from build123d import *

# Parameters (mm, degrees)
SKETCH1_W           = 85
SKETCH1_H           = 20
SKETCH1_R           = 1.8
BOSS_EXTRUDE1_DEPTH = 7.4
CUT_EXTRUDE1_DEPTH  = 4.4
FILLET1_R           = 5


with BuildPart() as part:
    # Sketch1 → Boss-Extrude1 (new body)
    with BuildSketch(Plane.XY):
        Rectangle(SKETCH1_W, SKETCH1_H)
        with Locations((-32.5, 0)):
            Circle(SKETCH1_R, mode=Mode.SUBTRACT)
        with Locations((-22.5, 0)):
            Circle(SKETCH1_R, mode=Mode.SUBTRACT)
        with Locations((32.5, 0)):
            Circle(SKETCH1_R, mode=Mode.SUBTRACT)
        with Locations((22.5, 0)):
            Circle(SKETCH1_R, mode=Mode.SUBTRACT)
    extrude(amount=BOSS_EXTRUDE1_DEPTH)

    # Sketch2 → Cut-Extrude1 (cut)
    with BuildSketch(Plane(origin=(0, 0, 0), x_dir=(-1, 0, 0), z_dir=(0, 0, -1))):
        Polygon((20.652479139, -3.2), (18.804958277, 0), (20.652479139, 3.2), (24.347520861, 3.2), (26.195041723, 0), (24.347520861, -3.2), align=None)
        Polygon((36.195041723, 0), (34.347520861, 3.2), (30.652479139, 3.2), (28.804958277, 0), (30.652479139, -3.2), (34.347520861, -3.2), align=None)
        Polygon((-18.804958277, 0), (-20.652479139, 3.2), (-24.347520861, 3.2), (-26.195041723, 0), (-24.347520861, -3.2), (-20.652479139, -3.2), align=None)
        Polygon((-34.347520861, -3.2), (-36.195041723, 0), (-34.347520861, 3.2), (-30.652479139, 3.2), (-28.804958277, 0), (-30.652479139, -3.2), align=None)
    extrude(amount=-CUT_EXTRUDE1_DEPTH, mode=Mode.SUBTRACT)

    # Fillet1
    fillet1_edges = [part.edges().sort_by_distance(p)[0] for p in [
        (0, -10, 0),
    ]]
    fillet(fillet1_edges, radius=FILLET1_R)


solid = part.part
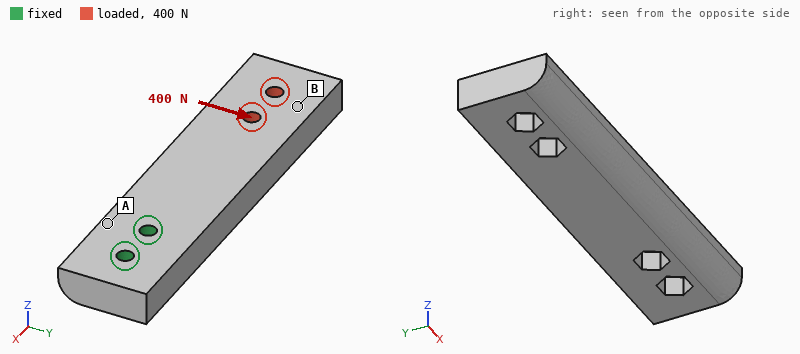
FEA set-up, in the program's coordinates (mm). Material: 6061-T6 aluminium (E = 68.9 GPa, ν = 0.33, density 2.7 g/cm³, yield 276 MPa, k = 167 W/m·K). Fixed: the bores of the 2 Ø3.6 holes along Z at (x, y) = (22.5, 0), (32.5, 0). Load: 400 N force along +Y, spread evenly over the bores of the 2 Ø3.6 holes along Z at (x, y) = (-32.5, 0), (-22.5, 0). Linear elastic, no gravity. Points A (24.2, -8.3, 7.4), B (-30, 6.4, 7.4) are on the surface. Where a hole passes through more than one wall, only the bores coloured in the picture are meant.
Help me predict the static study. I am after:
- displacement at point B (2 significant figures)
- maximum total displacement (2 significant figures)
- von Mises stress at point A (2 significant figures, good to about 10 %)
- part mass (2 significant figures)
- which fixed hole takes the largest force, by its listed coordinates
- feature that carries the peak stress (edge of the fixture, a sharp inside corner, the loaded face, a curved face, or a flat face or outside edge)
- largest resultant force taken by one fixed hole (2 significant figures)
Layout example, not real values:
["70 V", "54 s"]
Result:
["0.13 mm", "0.17 mm", "31 MPa", "31 g", "(22.5, 0)", "edge of the fixture", "1.8 kN"]
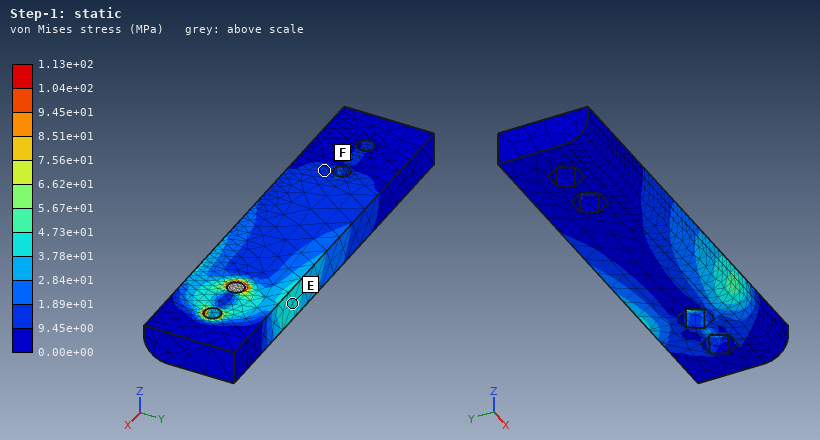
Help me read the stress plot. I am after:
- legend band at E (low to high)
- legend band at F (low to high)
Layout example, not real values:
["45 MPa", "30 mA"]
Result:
["3.78e+01 to 4.73e+01 MPa", "9.45e+00 to 1.89e+01 MPa"]
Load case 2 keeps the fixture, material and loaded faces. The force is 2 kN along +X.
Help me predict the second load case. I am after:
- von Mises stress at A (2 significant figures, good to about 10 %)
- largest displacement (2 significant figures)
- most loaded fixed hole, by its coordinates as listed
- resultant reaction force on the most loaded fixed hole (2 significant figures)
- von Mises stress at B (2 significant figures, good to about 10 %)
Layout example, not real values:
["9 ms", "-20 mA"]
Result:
["18 MPa", "0.19 mm", "(22.5, 0)", "1.5 kN", "17 MPa"]
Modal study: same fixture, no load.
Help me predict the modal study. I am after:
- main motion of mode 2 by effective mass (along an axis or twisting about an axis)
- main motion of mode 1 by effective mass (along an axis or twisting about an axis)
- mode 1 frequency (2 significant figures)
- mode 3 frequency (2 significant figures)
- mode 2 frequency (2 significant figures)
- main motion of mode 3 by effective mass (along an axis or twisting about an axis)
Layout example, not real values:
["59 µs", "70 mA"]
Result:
["along Y", "along Z", "1200 Hz", "6000 Hz", "2600 Hz", "twisting about X"]
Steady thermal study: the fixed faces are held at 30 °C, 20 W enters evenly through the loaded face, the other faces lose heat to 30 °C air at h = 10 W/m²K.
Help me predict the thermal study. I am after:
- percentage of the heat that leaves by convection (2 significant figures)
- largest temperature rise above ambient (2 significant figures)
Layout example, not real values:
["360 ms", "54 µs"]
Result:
["5.8 %", "50 K"]
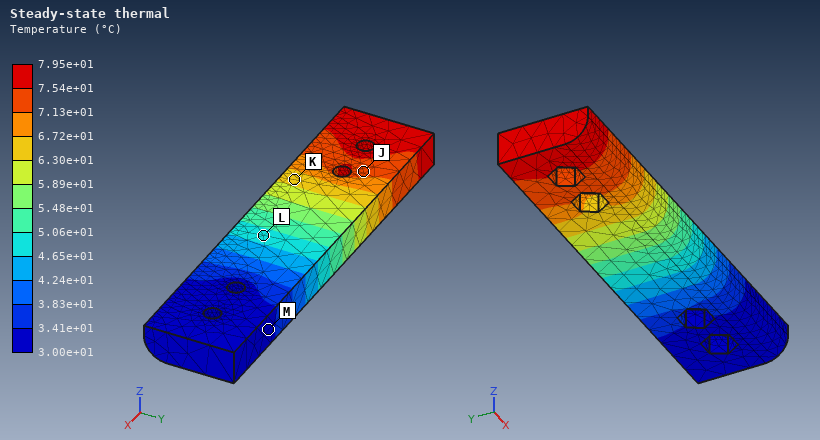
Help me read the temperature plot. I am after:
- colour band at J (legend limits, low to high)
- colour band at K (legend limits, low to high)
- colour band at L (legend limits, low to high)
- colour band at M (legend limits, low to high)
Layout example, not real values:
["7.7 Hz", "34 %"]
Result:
["7.13e+01 to 7.54e+01 °C", "6.30e+01 to 6.72e+01 °C", "4.65e+01 to 5.06e+01 °C", "3.00e+01 to 3.41e+01 °C"]
